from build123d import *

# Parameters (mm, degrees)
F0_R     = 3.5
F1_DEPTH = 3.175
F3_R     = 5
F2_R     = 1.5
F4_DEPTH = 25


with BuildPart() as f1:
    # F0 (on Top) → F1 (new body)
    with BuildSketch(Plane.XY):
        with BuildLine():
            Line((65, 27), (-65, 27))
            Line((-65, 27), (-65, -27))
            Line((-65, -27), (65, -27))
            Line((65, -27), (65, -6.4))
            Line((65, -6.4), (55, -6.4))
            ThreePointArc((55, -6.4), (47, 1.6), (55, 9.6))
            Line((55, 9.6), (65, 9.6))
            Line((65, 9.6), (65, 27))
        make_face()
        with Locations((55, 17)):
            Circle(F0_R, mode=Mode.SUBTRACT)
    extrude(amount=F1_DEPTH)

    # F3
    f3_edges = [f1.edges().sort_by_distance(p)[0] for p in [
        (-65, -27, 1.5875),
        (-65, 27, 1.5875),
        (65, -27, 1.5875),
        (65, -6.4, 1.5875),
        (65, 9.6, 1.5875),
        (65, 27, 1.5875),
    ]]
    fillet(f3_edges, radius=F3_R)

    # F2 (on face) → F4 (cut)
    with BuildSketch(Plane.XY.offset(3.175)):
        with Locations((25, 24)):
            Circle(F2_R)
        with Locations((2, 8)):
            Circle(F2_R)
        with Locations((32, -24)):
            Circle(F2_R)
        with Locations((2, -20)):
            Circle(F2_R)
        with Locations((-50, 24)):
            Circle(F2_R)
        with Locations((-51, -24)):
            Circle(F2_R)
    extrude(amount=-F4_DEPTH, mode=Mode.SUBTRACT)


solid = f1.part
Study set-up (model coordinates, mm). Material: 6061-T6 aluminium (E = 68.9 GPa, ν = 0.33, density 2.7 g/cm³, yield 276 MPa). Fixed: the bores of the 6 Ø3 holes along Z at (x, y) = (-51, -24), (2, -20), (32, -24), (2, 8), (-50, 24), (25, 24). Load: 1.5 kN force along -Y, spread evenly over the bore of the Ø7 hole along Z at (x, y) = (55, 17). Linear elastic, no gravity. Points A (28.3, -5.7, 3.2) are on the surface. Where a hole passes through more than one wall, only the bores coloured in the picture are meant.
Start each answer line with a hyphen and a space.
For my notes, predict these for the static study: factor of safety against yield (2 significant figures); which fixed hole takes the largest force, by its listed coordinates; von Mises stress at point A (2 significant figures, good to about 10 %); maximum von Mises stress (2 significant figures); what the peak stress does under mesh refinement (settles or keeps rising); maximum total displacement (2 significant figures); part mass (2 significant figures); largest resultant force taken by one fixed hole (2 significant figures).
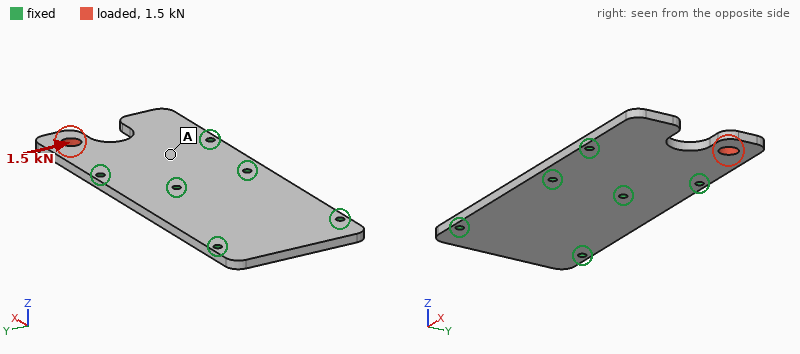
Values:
- 2.0
- (25, 24)
- 15 MPa
- 140 MPa
- settles
- 68 µm
- 57 g
- 1.1 kN
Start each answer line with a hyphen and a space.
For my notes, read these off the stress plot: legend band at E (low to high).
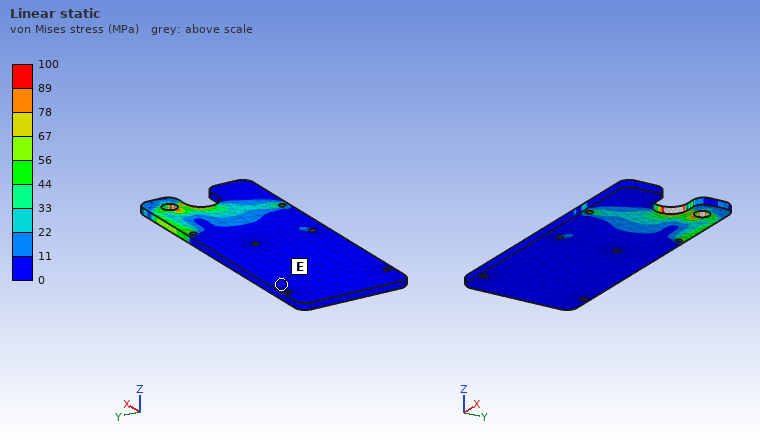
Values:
- 0 to 11 MPa
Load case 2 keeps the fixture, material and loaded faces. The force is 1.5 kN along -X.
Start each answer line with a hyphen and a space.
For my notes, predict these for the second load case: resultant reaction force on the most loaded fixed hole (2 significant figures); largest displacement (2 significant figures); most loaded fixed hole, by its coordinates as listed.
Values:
- 990 N
- 16 µm
- (25, 24)
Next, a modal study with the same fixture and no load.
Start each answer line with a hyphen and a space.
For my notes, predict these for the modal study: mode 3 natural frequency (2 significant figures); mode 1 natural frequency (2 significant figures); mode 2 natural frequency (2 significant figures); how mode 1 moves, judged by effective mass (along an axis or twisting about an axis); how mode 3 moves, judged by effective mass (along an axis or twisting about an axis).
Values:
- 4700 Hz
- 2000 Hz
- 2900 Hz
- along Z
- along Z
